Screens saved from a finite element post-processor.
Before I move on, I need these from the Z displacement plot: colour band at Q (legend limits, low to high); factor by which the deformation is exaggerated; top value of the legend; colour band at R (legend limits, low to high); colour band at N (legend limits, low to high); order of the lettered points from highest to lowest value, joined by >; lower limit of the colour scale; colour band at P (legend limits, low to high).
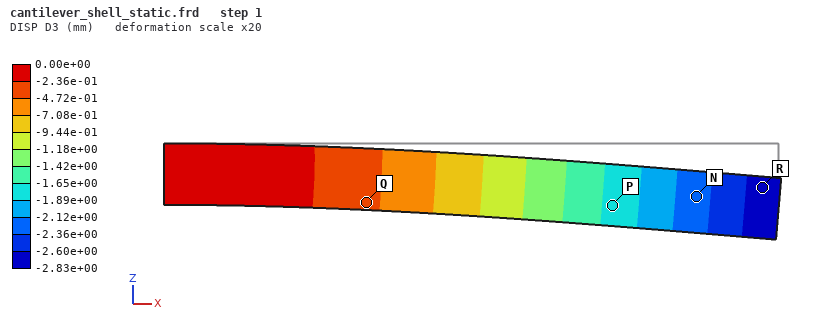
-4.72e-01 to -2.36e-01 mm
20
0.00e+00 mm
-2.83e+00 to -2.60e+00 mm
-2.36e+00 to -2.12e+00 mm
Q > P > N > R
-2.83e+00 mm
-1.89e+00 to -1.65e+00 mm
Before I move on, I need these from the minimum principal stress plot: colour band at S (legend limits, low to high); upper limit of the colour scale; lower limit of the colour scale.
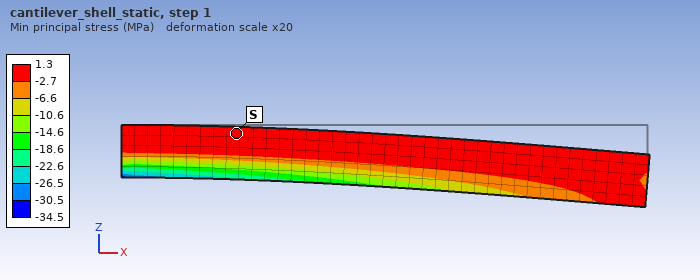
-2.7 to 1.3 MPa
1.3 MPa
-34.5 MPa
